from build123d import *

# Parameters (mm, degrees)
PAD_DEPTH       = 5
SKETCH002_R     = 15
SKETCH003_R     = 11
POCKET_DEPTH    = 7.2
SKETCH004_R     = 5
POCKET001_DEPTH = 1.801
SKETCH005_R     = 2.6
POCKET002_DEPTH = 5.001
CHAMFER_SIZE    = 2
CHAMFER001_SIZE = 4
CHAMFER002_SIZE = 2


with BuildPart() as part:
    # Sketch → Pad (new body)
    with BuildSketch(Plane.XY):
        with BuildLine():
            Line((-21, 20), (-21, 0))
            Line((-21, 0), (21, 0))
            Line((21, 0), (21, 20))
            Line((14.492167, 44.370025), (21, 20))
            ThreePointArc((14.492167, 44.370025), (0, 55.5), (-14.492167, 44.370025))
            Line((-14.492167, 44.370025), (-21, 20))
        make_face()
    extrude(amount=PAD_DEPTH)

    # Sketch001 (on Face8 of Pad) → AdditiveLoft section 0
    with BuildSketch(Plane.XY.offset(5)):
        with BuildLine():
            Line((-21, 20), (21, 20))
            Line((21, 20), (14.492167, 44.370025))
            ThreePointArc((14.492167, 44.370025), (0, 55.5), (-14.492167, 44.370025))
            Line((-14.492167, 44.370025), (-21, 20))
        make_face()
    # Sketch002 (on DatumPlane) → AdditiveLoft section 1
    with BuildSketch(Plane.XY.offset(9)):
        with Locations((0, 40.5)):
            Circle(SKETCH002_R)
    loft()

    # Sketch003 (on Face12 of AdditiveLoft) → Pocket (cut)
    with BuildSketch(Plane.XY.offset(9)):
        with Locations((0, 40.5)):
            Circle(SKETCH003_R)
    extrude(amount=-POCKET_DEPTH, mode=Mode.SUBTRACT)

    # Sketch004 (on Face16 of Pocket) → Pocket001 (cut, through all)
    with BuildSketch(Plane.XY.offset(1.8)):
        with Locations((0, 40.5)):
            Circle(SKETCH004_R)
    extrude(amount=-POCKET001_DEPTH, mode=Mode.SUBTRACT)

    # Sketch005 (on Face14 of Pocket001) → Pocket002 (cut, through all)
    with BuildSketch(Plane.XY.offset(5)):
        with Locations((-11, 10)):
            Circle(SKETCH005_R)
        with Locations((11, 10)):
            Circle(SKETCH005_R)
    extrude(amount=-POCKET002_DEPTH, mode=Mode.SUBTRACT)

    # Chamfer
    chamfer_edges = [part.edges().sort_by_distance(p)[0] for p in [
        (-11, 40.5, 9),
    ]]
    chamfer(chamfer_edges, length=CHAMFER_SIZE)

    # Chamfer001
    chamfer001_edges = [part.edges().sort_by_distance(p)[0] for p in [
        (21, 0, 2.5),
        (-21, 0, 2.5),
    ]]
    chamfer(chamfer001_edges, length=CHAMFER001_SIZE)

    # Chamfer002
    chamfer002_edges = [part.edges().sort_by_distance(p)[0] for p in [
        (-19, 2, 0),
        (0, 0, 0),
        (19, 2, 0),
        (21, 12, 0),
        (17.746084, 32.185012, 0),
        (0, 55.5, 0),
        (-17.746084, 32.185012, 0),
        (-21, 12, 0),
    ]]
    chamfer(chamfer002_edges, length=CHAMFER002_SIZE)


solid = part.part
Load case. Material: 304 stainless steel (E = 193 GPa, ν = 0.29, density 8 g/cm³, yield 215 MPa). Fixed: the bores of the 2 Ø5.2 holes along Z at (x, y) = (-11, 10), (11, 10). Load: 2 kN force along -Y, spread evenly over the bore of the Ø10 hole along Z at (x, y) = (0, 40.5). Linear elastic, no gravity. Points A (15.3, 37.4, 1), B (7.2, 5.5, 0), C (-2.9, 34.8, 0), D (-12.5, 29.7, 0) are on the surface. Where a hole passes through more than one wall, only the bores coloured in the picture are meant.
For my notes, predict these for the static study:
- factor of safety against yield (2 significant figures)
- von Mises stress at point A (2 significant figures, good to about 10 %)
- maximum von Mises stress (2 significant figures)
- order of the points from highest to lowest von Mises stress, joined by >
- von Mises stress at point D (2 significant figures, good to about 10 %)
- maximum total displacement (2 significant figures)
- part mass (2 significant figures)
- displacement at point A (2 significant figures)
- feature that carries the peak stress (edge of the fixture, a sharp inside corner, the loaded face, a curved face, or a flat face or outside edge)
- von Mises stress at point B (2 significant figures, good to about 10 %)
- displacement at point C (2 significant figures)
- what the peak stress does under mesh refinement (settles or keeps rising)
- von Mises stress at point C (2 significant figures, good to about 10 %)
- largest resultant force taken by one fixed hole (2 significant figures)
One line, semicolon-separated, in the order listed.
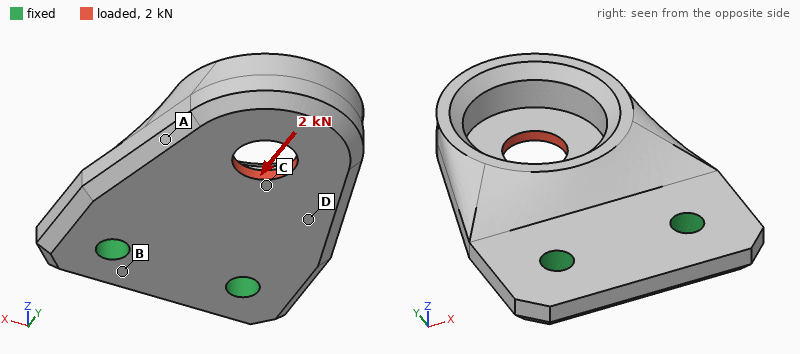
2.5; 14 MPa; 87 MPa; C > D > A > B; 24 MPa; 29 µm; 77 g; 12 µm; the loaded face; 7.3 MPa; 12 µm; settles; 44 MPa; 1.0 kN
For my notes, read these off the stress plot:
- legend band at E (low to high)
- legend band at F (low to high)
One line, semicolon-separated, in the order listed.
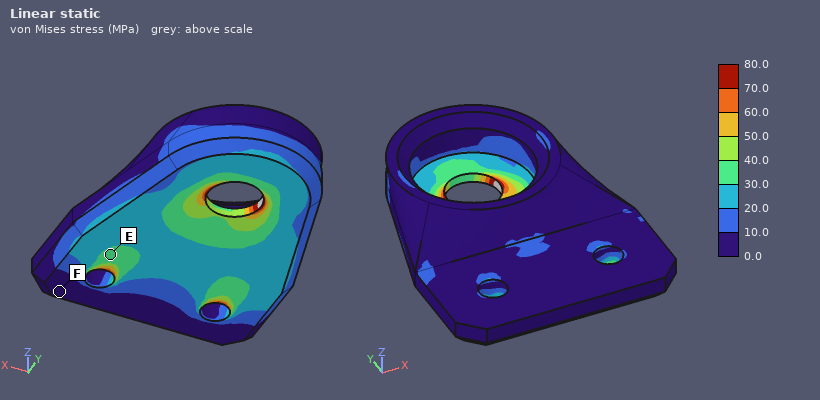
30.0 to 40.0 MPa; 0.0 to 10.0 MPa
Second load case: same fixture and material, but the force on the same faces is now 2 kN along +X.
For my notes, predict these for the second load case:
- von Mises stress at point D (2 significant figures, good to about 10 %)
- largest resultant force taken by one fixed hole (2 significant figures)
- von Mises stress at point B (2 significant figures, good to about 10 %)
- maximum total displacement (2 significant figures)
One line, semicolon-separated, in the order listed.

29 MPa; 2.5 kN; 12 MPa; 18 µm
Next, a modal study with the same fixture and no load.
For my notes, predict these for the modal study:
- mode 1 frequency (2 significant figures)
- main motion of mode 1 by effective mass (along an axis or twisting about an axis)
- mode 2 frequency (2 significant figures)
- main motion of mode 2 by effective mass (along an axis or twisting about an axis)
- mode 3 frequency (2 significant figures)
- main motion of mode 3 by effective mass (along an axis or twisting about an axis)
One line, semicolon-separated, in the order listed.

2800 Hz; along Z; 8100 Hz; twisting about Y; 11 kHz; along X
